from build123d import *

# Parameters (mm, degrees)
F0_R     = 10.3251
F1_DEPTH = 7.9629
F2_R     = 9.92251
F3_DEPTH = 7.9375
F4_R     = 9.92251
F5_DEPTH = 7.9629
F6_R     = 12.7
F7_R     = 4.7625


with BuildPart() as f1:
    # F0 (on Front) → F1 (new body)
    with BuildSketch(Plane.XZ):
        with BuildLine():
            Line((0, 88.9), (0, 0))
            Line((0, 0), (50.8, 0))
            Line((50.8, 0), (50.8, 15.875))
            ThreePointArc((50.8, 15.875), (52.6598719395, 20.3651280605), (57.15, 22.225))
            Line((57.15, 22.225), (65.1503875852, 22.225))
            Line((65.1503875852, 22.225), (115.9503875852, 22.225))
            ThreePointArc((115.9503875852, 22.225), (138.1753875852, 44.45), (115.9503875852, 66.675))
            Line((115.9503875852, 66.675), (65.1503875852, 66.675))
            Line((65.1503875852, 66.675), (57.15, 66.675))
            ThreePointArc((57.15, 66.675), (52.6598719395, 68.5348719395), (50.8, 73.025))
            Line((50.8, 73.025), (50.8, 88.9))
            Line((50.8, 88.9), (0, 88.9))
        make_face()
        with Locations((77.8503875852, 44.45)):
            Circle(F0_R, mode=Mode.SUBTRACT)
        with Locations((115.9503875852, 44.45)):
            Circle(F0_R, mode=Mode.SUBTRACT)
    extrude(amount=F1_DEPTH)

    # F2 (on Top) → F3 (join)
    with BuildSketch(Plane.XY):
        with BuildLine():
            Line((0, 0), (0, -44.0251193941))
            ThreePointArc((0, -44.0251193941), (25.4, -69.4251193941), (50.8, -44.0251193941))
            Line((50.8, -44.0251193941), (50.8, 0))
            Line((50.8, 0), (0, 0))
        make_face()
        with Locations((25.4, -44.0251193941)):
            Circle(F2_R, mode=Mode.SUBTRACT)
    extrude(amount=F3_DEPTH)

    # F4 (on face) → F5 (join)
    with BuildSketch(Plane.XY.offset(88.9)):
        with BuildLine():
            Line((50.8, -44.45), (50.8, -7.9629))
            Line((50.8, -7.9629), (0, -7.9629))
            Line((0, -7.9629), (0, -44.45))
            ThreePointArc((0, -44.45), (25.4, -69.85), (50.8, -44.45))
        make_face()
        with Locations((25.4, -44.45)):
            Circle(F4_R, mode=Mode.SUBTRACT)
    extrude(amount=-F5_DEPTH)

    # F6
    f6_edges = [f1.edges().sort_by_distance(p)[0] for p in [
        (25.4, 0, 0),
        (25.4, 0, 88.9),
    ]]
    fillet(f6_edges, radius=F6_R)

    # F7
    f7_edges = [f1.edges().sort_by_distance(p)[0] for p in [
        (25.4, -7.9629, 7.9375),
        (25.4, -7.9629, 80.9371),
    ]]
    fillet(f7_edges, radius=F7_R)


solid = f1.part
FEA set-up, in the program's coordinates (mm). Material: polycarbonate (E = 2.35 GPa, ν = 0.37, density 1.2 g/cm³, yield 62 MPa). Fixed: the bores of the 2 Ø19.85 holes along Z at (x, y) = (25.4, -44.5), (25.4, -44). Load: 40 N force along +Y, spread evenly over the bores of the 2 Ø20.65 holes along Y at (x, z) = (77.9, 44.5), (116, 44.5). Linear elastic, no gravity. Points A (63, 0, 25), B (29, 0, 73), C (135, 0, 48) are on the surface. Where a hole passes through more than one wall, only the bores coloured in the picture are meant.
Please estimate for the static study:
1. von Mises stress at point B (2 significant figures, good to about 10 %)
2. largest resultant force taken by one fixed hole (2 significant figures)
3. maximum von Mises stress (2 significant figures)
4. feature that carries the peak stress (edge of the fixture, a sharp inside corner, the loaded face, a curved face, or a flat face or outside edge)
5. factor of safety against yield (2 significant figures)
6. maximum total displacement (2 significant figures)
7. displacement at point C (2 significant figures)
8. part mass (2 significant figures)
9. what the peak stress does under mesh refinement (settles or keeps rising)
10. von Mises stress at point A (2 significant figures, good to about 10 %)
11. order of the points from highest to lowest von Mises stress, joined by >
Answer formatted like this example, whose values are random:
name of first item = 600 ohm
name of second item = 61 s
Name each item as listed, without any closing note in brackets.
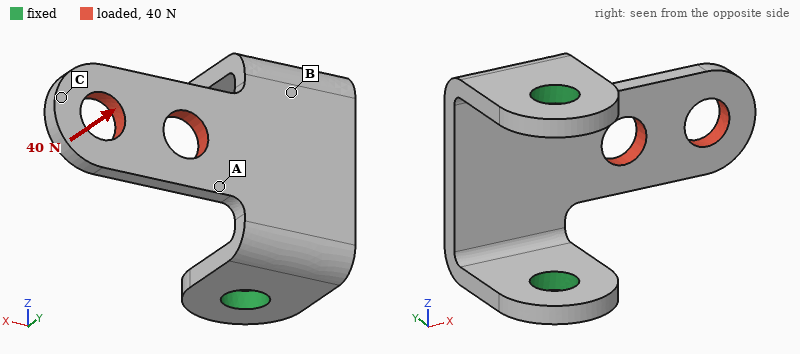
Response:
von Mises stress at point B = 1.5 MPa
largest resultant force taken by one fixed hole = 27 N
maximum von Mises stress = 6.1 MPa
feature that carries the peak stress = a curved face
factor of safety against yield = 10
maximum total displacement = 1.9 mm
displacement at point C = 1.8 mm
part mass = 120 g
what the peak stress does under mesh refinement = settles
von Mises stress at point A = 3.8 MPa
order of the points from highest to lowest von Mises stress, joined by > = A > B > C
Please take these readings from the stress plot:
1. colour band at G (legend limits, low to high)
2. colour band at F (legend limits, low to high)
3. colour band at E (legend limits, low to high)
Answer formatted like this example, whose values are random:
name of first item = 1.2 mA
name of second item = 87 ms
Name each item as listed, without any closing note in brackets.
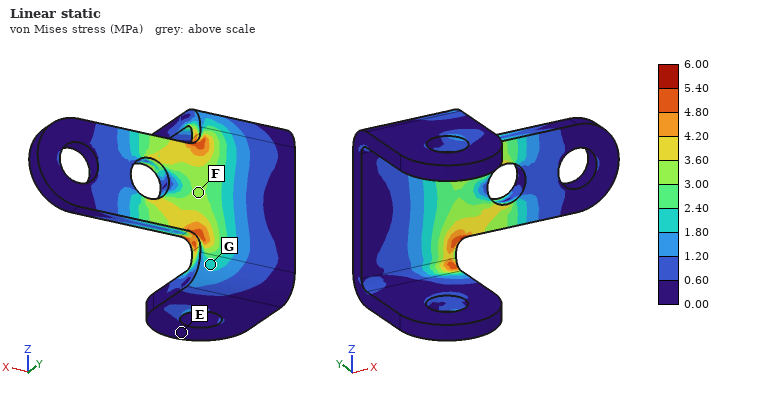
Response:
colour band at G = 1.80 to 2.40 MPa
colour band at F = 3.00 to 3.60 MPa
colour band at E = 0.00 to 0.60 MPa
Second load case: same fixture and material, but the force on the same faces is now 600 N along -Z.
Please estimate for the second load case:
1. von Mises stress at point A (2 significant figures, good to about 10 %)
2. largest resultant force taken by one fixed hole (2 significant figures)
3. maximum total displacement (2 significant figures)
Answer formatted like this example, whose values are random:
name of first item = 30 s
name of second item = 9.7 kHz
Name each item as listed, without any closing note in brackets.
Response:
von Mises stress at point A = 8.6 MPa
largest resultant force taken by one fixed hole = 600 N
maximum total displacement = 1.6 mm
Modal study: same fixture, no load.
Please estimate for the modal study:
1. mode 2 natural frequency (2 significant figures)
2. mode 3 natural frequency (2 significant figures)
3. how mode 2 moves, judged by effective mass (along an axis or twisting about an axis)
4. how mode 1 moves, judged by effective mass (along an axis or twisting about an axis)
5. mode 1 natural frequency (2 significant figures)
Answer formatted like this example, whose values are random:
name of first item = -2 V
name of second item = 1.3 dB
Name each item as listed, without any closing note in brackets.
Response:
mode 2 natural frequency = 640 Hz
mode 3 natural frequency = 800 Hz
how mode 2 moves, judged by effective mass = along Z
how mode 1 moves, judged by effective mass = along Y
mode 1 natural frequency = 180 Hz
